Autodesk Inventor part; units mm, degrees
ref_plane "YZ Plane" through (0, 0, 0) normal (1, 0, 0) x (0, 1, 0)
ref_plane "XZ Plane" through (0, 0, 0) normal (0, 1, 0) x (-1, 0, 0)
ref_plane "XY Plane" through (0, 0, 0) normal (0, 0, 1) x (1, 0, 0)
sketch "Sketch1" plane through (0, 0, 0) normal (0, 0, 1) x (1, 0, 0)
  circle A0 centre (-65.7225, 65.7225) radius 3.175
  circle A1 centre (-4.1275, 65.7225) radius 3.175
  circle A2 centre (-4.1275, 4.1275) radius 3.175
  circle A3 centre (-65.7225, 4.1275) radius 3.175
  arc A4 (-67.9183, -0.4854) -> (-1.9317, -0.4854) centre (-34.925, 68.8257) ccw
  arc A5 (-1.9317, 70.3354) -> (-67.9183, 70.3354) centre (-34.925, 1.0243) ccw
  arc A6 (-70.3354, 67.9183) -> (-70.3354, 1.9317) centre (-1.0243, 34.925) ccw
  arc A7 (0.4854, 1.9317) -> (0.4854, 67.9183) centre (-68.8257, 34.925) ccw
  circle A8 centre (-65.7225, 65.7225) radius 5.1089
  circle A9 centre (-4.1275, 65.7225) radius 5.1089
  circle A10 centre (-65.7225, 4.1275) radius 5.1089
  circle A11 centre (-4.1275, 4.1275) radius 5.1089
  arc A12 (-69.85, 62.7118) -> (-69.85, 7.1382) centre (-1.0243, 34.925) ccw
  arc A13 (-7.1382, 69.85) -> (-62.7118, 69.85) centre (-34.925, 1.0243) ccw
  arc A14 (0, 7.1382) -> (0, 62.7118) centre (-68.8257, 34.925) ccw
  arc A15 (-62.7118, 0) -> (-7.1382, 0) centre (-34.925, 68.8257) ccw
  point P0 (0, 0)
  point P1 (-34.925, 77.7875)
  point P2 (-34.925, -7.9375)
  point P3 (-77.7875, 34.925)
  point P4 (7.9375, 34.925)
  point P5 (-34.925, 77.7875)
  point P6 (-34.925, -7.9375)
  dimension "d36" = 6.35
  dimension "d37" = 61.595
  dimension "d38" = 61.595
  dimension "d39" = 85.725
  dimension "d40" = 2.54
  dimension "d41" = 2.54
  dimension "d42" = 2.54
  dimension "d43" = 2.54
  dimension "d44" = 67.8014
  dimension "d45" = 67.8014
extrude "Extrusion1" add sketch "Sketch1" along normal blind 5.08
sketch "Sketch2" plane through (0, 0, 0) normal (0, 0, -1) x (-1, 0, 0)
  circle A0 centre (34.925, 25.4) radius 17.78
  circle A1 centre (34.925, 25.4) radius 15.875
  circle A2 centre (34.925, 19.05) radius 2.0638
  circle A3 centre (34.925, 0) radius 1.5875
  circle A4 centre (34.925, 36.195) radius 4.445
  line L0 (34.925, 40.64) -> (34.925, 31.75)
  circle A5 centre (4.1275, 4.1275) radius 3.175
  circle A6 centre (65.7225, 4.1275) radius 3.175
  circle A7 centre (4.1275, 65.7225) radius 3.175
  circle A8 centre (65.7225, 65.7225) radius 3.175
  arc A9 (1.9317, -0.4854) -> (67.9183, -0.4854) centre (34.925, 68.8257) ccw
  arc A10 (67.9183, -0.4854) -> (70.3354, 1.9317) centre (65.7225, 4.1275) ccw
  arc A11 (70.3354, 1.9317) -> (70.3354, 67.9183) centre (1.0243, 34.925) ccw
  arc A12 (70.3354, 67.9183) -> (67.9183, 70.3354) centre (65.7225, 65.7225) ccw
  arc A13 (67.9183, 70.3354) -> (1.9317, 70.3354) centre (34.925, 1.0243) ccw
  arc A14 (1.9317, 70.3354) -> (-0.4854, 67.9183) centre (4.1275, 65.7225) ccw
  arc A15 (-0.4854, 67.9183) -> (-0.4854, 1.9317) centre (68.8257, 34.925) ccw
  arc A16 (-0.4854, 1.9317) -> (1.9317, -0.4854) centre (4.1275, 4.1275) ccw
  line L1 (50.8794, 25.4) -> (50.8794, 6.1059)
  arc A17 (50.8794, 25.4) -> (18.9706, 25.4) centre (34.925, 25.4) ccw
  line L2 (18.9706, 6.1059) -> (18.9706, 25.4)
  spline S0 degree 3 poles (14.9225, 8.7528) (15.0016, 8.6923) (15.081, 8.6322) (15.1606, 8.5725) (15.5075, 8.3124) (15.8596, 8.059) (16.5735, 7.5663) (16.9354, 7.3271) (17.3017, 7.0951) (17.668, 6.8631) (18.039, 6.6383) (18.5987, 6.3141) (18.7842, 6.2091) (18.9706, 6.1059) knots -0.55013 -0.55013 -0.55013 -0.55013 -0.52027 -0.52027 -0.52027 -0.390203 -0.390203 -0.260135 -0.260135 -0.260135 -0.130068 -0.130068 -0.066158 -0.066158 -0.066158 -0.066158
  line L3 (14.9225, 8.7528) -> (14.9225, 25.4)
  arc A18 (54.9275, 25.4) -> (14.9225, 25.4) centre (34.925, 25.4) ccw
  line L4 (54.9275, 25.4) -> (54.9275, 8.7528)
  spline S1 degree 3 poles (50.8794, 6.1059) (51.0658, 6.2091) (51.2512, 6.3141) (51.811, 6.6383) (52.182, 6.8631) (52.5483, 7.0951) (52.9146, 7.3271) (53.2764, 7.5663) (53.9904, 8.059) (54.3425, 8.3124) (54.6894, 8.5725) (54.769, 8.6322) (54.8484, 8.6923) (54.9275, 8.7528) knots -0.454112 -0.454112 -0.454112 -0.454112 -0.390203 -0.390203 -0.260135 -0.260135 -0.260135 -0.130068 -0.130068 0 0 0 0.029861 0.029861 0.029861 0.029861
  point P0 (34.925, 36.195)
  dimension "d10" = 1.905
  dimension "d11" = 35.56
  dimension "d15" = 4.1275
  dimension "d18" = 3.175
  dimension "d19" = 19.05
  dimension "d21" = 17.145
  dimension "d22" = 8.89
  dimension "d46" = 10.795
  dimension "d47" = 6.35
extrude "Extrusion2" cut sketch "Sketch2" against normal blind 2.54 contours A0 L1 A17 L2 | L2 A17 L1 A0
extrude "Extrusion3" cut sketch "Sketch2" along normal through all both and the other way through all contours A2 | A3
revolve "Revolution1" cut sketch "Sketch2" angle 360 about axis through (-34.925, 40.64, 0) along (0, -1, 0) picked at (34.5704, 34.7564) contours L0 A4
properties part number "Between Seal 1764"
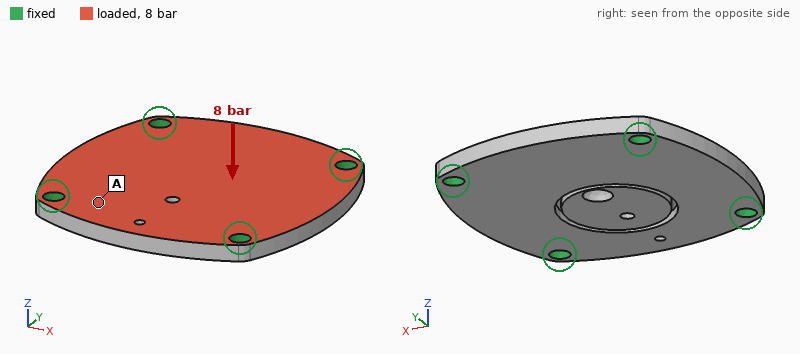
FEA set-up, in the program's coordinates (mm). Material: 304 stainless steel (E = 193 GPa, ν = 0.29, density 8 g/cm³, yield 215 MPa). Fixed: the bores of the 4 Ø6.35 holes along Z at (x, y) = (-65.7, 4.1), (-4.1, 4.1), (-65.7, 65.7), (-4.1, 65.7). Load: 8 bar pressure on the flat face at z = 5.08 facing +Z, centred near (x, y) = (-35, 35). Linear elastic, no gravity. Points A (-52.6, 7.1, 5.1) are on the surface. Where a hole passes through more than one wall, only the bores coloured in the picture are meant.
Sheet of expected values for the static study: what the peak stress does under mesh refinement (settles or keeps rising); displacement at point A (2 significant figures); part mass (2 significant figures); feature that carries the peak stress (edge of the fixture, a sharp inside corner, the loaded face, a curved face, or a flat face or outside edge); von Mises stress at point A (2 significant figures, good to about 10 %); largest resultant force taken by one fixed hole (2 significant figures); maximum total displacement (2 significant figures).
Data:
keeps rising
11 µm
250 g
edge of the fixture
22 MPa
1.3 kN
38 µm
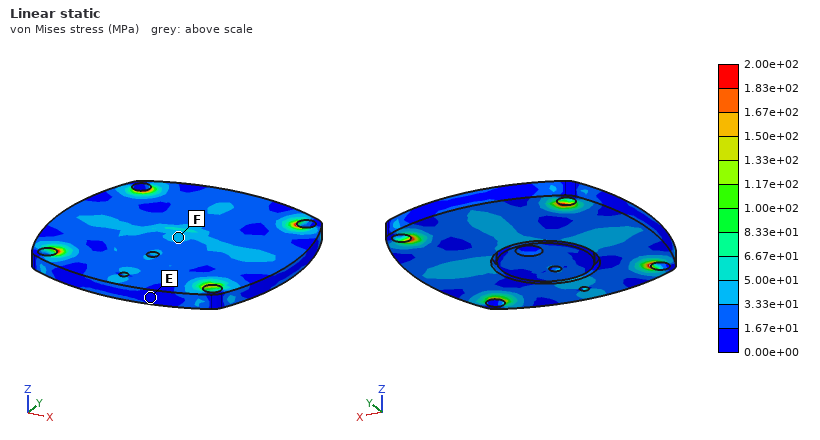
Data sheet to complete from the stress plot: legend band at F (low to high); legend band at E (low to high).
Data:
3.33e+01 to 5.00e+01 MPa
0.00e+00 to 1.67e+01 MPa
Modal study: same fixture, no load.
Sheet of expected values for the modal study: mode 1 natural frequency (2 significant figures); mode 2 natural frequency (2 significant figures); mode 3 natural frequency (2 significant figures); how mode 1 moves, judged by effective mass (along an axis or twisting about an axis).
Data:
4700 Hz
6900 Hz
7000 Hz
along Z
